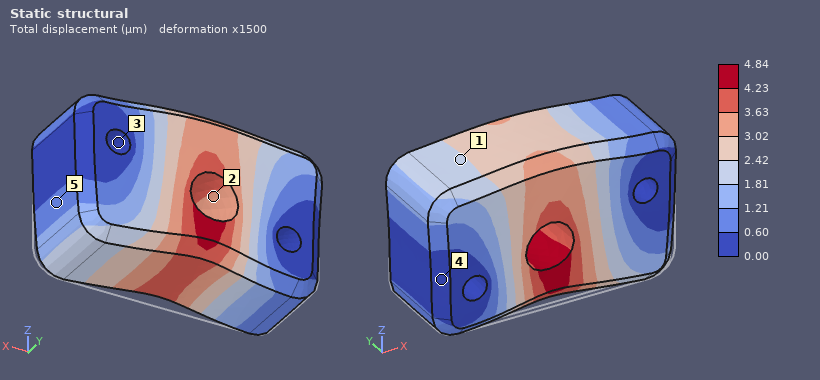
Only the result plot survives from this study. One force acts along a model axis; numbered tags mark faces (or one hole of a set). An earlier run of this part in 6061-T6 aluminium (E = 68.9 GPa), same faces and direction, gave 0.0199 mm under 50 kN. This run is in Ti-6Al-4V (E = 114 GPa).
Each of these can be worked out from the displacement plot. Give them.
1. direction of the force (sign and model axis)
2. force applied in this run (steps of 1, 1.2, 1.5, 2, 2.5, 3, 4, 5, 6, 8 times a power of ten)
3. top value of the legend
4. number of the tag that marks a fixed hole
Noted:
+Z
20 kN
4.84 µm
3
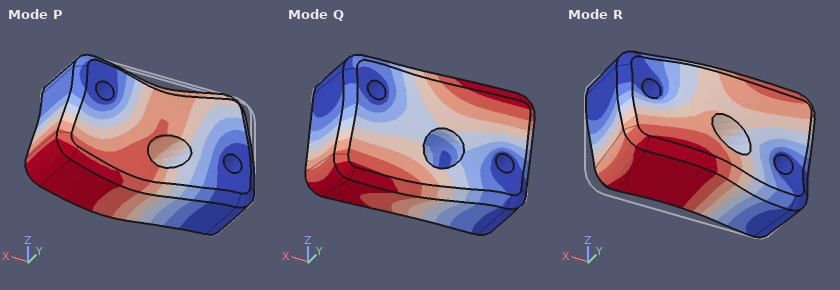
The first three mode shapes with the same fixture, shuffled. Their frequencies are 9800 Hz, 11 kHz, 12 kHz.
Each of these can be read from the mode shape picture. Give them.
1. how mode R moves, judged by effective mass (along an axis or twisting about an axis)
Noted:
along Y
